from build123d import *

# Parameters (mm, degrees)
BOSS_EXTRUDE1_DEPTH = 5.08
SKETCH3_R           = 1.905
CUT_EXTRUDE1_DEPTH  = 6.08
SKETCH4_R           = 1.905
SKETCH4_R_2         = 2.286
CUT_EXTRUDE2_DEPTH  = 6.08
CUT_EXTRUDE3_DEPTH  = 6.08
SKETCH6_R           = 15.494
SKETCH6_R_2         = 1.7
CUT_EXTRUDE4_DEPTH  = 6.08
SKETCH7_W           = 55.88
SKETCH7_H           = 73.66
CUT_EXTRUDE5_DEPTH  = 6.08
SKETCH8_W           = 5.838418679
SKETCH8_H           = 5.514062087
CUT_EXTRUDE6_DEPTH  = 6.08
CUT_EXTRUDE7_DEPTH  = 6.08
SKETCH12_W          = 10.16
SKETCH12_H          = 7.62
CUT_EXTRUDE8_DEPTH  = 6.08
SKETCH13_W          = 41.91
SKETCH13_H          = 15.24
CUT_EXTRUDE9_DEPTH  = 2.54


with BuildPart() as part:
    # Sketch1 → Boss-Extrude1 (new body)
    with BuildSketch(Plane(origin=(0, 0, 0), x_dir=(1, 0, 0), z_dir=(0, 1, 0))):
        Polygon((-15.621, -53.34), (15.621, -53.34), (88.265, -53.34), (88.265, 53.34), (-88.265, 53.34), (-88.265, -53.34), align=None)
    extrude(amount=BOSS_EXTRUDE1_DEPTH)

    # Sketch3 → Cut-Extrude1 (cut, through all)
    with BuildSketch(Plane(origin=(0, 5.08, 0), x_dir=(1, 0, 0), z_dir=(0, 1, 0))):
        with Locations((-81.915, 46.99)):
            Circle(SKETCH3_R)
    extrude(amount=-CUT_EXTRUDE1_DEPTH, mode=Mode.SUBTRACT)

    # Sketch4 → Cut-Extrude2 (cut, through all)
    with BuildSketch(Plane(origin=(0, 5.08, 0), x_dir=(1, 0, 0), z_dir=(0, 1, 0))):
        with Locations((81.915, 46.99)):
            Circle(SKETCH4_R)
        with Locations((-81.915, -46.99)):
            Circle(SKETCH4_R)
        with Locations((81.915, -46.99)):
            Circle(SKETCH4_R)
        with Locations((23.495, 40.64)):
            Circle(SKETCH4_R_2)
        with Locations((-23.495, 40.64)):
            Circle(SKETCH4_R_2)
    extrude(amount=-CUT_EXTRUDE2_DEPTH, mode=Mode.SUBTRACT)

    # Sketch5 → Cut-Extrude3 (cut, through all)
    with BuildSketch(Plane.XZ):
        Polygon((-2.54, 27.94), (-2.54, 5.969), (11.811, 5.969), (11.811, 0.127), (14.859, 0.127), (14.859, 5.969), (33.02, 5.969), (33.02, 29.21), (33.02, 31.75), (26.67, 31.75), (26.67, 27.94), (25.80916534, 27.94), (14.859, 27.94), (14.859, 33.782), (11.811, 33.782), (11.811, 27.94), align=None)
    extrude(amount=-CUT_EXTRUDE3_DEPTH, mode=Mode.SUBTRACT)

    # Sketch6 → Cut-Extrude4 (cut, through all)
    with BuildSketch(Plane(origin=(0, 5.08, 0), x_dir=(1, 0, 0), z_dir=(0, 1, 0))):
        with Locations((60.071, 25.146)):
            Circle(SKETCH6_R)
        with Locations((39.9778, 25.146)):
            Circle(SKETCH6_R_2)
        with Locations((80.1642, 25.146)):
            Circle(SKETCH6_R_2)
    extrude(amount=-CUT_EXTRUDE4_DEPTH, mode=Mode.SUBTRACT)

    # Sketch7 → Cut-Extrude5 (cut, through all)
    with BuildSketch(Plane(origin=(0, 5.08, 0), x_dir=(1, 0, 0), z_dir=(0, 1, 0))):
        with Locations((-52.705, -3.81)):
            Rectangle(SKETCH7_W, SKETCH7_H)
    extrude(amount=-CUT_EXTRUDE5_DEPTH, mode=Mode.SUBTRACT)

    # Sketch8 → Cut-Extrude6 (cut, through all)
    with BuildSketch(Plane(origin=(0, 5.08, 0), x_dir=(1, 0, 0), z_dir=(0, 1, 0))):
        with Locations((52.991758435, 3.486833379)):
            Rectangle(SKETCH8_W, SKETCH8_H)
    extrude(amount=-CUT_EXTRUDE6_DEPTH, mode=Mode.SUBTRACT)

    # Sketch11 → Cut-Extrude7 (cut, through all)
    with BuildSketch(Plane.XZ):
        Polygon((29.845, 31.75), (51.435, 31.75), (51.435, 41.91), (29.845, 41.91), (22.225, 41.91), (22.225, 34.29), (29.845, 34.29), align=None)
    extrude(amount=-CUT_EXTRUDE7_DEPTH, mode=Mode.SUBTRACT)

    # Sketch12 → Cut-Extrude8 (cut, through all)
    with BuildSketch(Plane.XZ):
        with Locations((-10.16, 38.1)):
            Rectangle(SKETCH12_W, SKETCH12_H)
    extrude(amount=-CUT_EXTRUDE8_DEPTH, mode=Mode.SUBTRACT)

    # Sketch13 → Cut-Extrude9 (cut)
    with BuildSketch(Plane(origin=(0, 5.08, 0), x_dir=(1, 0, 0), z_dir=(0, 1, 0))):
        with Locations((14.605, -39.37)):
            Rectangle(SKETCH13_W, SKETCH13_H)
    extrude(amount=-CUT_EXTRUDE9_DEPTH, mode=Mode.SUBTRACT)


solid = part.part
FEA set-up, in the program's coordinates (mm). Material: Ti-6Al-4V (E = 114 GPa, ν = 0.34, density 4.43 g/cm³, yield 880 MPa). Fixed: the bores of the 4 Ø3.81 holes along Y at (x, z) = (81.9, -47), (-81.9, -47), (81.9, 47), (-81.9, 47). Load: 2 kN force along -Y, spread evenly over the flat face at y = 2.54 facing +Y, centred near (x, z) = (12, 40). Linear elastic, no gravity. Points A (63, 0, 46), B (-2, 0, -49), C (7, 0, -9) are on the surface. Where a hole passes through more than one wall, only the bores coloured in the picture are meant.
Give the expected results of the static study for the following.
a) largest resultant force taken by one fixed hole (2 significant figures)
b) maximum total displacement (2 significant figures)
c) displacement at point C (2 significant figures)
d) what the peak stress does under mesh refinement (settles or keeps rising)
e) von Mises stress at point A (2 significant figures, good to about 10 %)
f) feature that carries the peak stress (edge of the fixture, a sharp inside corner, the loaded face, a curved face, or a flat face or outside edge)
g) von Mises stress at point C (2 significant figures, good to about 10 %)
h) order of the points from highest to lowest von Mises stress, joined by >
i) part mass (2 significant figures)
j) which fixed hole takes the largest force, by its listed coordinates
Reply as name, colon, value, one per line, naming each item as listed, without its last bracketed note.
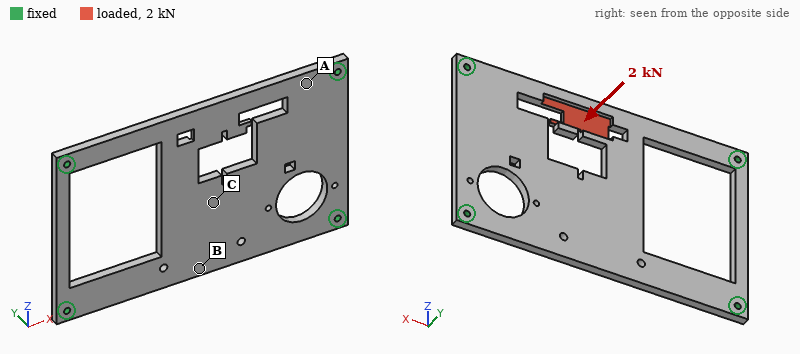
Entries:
largest resultant force taken by one fixed hole: 1.5 kN
maximum total displacement: 1.7 mm
displacement at point C: 0.66 mm
what the peak stress does under mesh refinement: keeps rising
von Mises stress at point A: 200 MPa
feature that carries the peak stress: edge of the fixture
von Mises stress at point C: 100 MPa
order of the points from highest to lowest von Mises stress, joined by >: A > C > B
part mass: 280 g
which fixed hole takes the largest force, by its listed coordinates: (81.9, 47)
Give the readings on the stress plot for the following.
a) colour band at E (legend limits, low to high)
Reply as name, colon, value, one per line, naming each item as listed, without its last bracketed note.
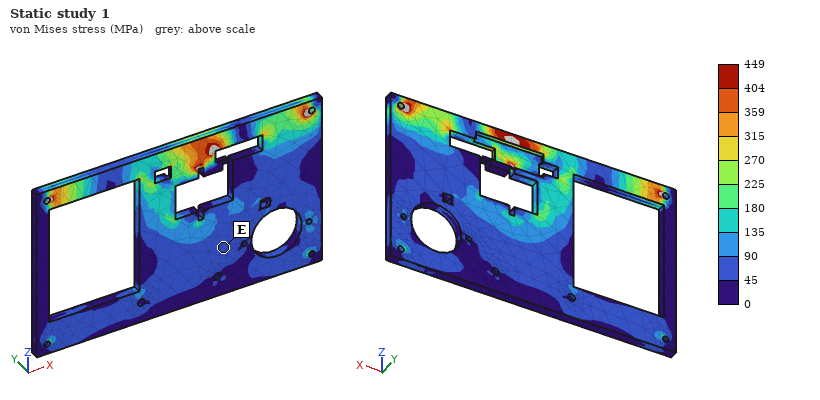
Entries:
colour band at E: 45 to 90 MPa
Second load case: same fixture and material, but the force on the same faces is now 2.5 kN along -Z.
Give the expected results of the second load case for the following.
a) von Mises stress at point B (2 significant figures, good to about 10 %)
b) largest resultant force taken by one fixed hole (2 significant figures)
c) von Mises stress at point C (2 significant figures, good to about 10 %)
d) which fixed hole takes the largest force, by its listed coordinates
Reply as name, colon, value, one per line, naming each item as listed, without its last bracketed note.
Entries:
von Mises stress at point B: 9.8 MPa
largest resultant force taken by one fixed hole: 2.0 kN
von Mises stress at point C: 15 MPa
which fixed hole takes the largest force, by its listed coordinates: (81.9, 47)
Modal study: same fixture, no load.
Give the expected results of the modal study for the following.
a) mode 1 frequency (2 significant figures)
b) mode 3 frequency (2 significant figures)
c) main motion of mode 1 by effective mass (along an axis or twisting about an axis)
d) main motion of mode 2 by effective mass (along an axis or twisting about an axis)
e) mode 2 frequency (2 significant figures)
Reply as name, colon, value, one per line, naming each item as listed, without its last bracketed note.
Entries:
mode 1 frequency: 710 Hz
mode 3 frequency: 1900 Hz
main motion of mode 1 by effective mass: along Y
main motion of mode 2 by effective mass: twisting about X
mode 2 frequency: 1100 Hz
